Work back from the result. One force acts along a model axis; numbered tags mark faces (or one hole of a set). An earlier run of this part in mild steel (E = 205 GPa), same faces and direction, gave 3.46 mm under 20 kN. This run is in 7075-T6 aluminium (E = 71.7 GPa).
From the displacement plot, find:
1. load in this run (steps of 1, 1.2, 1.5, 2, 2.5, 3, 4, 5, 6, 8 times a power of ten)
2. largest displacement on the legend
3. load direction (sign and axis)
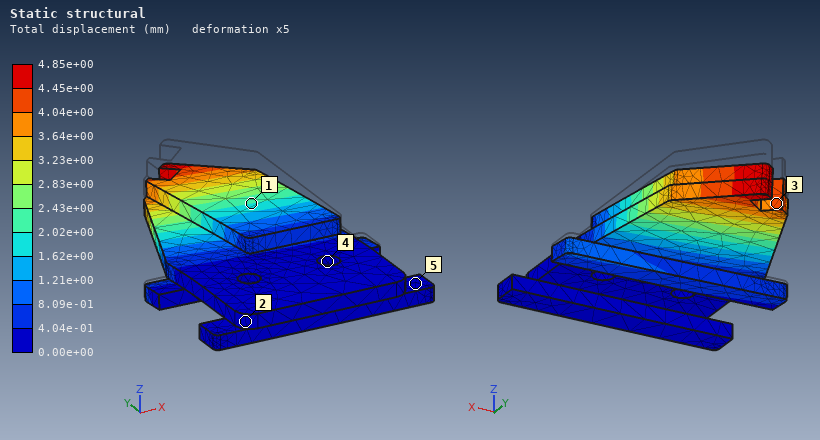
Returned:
10 kN
4.85e+00 mm
-Z
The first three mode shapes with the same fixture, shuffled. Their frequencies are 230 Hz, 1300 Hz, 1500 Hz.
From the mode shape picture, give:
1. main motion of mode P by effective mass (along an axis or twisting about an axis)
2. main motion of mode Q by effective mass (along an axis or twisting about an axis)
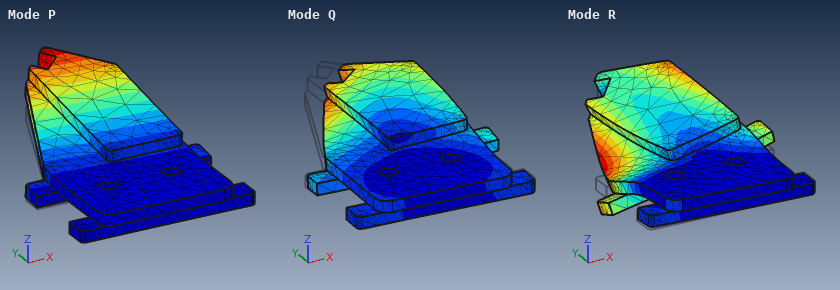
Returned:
along Z
along X
